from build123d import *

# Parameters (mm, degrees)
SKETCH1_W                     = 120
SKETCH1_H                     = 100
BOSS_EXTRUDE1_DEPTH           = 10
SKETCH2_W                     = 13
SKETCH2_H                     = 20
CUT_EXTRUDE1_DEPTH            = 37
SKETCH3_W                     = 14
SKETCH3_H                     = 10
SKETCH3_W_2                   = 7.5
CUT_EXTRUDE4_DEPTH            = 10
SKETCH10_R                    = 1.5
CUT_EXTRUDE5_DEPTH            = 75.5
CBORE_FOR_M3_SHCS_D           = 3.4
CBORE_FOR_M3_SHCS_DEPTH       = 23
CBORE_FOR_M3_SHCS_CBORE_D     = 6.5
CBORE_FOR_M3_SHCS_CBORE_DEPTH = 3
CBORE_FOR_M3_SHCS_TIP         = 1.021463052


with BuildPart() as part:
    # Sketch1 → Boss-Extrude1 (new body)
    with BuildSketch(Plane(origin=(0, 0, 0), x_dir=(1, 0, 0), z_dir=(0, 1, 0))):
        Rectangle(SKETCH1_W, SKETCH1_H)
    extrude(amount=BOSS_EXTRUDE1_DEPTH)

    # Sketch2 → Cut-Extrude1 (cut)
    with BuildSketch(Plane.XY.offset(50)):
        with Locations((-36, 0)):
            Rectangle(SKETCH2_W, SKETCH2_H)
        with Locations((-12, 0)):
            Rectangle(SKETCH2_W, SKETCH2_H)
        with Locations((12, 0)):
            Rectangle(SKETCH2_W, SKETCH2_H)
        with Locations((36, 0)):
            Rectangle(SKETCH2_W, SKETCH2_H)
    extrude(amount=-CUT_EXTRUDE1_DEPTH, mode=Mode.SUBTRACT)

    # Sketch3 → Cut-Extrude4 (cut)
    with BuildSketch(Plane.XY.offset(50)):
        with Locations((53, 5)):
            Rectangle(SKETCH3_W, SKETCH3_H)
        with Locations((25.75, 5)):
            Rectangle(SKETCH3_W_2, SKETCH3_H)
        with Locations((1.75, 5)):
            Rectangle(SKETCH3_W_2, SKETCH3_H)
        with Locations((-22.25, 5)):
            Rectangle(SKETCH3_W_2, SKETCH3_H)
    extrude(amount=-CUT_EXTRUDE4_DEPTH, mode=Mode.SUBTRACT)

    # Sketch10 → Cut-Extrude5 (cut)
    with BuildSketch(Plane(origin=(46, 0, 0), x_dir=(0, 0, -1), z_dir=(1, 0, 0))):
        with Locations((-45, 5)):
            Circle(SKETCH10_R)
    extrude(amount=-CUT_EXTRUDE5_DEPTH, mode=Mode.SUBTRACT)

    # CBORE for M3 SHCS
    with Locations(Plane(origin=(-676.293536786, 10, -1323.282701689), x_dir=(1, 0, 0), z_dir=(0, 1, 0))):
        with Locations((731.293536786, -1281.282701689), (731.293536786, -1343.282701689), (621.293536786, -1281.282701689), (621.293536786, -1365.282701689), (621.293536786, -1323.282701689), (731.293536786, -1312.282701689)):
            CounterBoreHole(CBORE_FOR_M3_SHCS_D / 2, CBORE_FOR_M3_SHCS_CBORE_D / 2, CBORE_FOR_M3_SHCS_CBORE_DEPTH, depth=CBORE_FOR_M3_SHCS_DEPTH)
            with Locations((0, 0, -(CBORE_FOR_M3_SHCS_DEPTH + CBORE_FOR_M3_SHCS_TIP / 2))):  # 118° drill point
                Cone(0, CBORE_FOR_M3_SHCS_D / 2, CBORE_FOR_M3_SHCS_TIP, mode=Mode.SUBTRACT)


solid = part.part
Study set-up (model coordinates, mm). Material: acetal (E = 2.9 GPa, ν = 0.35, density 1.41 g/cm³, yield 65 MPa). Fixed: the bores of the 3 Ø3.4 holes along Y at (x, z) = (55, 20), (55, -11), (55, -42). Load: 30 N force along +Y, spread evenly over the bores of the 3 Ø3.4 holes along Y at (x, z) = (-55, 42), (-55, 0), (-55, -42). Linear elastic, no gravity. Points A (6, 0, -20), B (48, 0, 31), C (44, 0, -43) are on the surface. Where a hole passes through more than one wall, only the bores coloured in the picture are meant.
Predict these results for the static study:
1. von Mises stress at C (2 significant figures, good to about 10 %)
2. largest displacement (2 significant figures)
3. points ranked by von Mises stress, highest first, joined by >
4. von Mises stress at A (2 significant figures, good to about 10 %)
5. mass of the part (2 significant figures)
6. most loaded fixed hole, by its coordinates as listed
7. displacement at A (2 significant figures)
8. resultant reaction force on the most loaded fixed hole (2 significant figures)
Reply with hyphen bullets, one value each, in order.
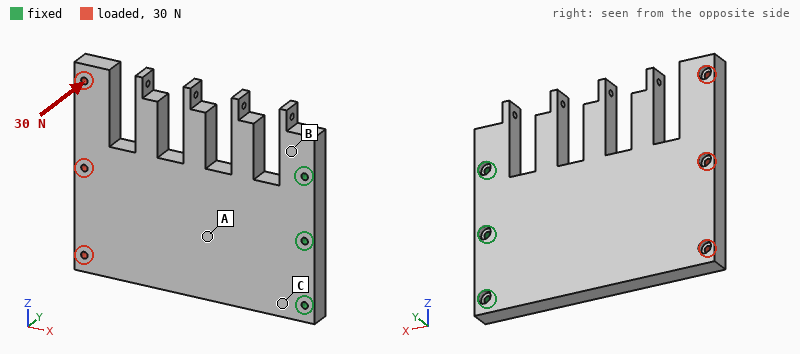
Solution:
- 2.9 MPa
- 1.5 mm
- C > A > B
- 1.7 MPa
- 140 g
- (55, -11)
- 0.36 mm
- 36 N
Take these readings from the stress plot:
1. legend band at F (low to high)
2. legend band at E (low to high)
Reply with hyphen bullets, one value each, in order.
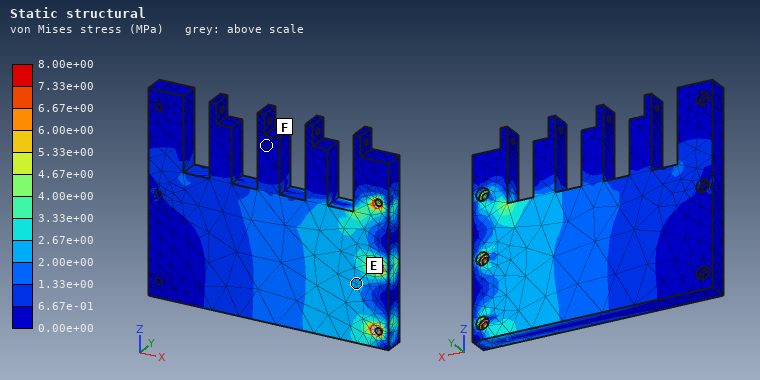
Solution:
- 0.00e+00 to 6.67e-01 MPa
- 2.00e+00 to 2.67e+00 MPa
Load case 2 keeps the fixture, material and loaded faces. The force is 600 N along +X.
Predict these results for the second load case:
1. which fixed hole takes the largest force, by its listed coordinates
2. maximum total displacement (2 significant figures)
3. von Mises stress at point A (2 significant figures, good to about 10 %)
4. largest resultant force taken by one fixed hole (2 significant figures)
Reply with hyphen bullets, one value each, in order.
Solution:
- (55, -11)
- 0.80 mm
- 1.7 MPa
- 370 N
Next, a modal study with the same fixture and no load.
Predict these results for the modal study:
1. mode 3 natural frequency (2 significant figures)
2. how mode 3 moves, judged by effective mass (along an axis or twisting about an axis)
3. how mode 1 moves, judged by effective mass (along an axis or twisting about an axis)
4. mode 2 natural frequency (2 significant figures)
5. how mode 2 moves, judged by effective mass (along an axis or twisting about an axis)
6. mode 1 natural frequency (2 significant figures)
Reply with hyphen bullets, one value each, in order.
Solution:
- 680 Hz
- along Z
- along Y
- 370 Hz
- twisting about X
- 130 Hz
